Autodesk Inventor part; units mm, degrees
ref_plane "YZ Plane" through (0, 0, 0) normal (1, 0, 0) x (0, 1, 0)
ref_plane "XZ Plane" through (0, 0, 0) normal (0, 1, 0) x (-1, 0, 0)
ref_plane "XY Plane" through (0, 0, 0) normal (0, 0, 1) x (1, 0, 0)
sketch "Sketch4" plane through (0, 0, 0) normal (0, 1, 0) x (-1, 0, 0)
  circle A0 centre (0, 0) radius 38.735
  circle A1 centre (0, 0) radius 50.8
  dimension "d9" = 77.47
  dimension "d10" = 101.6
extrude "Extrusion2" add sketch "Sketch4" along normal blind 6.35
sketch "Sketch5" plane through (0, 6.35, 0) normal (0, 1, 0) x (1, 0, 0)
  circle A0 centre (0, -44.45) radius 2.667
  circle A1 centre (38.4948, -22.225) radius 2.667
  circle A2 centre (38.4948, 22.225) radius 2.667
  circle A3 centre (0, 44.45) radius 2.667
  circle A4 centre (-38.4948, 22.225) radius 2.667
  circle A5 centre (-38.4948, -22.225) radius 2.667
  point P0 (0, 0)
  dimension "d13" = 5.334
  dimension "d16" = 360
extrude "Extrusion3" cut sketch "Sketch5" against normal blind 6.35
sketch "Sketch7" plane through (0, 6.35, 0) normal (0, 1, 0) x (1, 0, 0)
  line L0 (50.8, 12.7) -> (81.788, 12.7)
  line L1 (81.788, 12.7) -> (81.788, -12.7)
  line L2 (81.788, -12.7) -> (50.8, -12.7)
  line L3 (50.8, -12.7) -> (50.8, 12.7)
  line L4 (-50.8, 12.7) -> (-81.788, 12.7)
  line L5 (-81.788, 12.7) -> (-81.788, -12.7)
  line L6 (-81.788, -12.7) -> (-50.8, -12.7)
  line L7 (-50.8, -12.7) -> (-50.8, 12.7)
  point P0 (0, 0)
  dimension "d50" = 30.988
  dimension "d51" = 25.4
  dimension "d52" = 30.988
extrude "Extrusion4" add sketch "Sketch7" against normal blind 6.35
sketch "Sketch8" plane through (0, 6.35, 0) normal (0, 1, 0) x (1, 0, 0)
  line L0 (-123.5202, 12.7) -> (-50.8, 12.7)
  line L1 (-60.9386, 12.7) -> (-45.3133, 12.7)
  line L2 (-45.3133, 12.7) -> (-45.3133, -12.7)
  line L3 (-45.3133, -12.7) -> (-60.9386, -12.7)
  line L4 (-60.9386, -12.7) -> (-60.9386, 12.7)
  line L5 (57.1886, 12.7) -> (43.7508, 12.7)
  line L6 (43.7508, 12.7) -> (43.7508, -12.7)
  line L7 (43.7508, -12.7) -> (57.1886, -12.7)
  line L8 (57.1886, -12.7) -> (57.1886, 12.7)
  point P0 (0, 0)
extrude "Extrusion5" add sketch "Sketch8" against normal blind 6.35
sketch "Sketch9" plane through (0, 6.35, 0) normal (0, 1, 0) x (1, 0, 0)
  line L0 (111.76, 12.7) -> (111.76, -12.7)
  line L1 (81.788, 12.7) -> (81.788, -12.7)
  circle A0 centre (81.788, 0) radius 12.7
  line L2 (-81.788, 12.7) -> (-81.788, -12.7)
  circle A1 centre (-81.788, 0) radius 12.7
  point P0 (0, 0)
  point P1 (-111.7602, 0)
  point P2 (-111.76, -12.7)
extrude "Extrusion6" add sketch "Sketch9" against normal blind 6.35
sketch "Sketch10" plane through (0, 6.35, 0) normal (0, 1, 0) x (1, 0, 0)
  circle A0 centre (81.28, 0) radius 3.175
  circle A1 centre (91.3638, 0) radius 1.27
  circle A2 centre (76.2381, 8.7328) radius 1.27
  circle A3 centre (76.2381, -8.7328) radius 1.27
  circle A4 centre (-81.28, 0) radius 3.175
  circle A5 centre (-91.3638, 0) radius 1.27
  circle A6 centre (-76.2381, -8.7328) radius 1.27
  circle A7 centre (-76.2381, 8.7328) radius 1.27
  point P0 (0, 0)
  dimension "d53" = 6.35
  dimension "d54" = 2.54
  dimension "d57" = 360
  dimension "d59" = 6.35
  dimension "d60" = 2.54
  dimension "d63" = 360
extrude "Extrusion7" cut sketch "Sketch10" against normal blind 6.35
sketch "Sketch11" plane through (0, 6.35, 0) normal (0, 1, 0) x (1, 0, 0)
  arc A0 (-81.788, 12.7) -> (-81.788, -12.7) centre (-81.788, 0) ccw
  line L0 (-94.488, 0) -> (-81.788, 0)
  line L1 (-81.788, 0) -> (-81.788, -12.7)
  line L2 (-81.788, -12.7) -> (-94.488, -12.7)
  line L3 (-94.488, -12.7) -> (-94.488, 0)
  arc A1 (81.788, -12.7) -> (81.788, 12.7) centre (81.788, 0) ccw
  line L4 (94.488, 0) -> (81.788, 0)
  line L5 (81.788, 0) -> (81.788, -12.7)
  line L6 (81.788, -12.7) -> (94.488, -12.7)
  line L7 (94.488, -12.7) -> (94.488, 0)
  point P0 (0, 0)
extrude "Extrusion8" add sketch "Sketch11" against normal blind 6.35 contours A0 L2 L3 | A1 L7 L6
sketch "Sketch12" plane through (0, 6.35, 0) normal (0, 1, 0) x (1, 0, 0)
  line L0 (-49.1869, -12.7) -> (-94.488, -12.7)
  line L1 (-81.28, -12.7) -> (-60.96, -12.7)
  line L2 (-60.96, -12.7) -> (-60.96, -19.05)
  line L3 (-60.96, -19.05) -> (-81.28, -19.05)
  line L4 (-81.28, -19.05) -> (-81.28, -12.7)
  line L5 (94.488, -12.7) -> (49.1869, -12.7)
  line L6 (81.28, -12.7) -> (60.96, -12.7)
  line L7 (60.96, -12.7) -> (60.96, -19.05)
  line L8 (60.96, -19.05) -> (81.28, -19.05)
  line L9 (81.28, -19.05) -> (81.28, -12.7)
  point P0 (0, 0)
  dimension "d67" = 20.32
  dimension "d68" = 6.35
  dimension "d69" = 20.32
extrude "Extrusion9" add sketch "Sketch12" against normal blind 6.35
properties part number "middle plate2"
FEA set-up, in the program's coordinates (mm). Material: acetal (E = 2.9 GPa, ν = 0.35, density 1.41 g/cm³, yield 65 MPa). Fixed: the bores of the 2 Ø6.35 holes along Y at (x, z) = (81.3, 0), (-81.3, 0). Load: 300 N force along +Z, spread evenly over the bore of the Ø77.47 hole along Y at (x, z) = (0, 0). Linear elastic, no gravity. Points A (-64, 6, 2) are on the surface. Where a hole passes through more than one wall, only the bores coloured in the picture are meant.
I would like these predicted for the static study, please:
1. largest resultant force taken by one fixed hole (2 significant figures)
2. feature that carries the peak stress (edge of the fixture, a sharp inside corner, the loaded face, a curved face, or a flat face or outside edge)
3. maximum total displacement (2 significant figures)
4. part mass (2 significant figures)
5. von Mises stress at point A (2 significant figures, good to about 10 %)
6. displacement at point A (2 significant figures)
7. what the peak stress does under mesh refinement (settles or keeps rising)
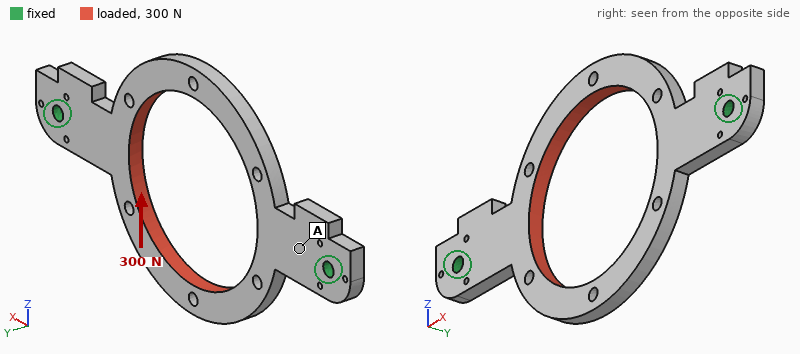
150 N
edge of the fixture
0.18 mm
50 g
2.1 MPa
0.075 mm
keeps rising
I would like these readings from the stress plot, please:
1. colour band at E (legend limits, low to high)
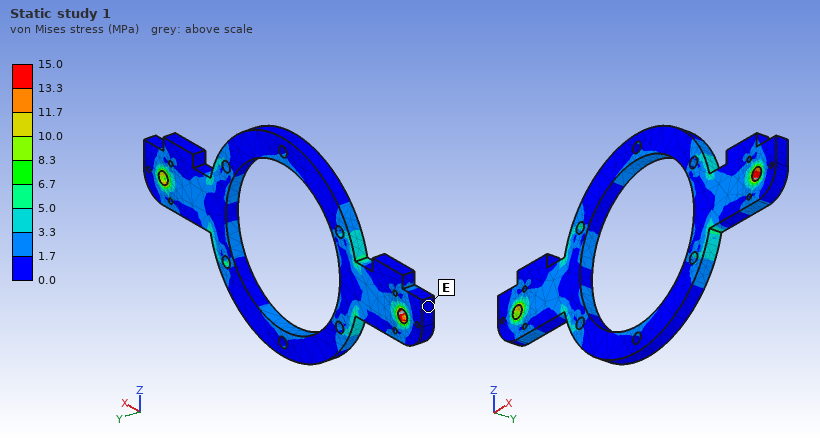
0.0 to 1.7 MPa
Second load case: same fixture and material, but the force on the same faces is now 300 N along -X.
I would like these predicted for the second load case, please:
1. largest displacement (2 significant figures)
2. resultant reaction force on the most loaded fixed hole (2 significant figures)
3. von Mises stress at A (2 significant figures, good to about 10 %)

87 µm
150 N
0.97 MPa
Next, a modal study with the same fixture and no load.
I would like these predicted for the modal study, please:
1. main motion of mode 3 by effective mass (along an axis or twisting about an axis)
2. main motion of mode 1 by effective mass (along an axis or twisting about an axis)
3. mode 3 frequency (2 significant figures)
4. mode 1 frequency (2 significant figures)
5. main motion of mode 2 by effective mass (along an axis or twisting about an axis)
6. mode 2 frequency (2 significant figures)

twisting about Z
twisting about X
690 Hz
260 Hz
along Y
280 Hz
